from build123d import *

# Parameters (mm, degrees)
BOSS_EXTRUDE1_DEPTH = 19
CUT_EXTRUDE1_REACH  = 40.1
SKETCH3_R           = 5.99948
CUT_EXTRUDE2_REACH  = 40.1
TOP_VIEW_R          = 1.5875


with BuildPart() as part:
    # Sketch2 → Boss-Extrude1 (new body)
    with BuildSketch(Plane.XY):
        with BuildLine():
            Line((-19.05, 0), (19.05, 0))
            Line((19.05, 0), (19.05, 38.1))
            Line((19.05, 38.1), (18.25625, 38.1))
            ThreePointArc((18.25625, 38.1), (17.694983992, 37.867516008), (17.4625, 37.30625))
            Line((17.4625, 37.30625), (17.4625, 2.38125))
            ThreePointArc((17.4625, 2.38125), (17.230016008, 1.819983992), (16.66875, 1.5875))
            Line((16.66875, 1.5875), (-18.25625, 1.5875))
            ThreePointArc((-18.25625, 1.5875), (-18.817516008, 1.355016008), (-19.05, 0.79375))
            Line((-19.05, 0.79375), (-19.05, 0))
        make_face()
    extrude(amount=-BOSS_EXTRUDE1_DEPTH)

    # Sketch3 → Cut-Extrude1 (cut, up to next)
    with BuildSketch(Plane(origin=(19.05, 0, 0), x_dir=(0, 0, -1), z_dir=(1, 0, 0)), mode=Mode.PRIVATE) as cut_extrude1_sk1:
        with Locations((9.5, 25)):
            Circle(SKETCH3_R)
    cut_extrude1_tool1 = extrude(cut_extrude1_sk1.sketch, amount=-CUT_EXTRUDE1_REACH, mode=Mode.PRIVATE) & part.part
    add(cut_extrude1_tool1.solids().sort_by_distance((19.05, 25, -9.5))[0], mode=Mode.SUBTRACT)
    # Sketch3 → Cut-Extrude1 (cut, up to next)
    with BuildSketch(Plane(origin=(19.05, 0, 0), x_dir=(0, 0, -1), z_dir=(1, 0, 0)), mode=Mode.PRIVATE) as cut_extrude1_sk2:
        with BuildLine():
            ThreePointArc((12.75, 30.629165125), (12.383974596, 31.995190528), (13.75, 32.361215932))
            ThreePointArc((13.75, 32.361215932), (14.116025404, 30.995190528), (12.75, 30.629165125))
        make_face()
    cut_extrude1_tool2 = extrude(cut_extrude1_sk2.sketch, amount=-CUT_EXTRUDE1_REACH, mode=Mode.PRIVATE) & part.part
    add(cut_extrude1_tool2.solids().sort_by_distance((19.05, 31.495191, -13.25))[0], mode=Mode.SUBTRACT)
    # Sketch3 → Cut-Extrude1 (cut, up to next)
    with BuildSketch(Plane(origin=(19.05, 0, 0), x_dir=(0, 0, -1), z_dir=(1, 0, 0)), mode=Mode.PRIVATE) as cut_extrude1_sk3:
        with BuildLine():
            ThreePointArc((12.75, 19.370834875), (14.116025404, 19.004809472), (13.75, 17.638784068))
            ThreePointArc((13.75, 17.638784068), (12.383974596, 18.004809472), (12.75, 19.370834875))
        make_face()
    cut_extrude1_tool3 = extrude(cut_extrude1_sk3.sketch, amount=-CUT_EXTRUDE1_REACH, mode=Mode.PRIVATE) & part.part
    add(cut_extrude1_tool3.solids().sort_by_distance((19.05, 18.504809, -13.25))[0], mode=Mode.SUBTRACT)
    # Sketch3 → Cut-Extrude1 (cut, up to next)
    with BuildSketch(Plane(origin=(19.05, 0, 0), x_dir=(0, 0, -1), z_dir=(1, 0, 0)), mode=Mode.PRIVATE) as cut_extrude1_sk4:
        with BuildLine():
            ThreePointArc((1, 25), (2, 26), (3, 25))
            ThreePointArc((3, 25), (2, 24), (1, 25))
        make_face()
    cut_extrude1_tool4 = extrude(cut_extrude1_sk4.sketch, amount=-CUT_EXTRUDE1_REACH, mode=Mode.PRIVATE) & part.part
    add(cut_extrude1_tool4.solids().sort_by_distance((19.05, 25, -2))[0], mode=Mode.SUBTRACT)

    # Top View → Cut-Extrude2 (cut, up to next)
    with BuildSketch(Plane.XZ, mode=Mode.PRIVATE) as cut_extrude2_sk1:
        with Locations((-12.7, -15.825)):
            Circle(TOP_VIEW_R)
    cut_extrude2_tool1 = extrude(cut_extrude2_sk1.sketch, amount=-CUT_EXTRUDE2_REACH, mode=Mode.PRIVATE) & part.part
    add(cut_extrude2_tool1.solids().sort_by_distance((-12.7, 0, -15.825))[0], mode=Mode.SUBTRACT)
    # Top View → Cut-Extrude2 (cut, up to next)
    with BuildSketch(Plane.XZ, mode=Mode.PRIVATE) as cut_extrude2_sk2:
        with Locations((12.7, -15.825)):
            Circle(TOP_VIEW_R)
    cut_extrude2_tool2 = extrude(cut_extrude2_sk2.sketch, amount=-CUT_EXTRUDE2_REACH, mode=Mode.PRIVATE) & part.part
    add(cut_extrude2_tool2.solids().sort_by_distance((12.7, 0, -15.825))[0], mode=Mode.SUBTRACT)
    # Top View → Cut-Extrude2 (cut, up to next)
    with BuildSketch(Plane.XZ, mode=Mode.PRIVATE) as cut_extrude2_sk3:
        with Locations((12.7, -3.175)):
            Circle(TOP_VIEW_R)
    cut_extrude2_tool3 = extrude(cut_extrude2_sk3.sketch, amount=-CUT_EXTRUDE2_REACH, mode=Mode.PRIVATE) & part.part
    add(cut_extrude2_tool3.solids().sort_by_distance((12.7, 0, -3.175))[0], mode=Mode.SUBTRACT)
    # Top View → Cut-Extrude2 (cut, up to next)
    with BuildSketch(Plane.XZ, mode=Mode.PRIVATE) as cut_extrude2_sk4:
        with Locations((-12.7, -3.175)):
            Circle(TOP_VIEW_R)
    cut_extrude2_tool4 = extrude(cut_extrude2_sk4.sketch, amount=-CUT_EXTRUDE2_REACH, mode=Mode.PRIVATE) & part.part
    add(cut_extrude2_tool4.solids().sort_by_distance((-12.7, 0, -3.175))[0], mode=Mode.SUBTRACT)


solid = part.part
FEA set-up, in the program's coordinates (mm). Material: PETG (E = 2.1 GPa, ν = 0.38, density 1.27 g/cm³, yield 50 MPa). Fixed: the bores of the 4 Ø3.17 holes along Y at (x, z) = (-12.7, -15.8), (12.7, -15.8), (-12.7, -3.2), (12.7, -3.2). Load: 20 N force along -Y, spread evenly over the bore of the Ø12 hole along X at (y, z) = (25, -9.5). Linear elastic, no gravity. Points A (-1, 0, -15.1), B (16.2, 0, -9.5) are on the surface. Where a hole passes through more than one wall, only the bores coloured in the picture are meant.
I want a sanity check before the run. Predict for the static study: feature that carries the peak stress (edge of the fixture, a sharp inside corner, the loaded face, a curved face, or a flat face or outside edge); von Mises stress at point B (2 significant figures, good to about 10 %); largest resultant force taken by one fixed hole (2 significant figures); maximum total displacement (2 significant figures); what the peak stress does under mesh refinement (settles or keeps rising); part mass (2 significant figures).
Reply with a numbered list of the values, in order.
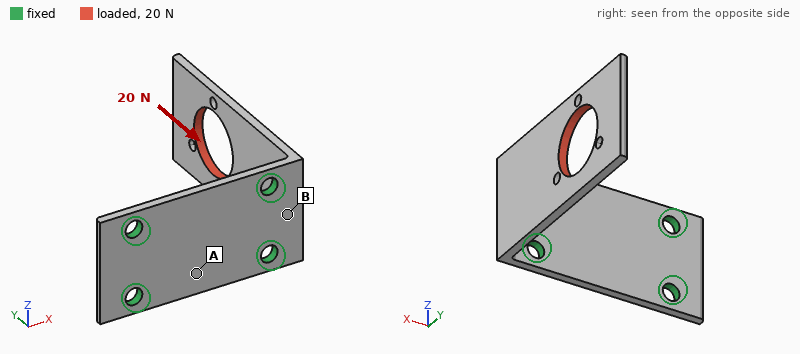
1. edge of the fixture
2. 3.3 MPa
3. 10 N
4. 0.57 mm
5. keeps rising
6. 2.5 g
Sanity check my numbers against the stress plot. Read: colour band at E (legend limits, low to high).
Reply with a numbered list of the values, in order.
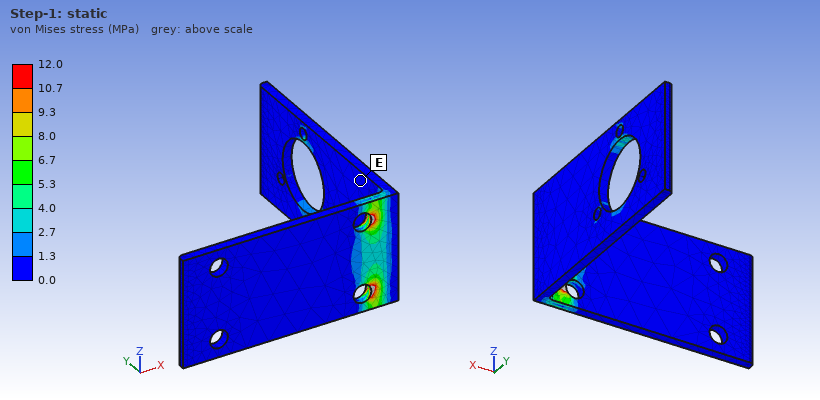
1. 0.0 to 1.3 MPa
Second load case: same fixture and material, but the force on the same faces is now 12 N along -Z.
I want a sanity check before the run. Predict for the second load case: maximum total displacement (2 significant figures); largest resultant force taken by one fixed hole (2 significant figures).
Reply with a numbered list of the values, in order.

1. 0.55 mm
2. 23 N
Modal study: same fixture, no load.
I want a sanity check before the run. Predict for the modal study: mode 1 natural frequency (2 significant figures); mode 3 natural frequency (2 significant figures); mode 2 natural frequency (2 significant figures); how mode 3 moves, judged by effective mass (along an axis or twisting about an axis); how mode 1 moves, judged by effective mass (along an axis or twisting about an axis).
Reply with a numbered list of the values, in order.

1. 230 Hz
2. 1100 Hz
3. 820 Hz
4. along Z
5. along X
